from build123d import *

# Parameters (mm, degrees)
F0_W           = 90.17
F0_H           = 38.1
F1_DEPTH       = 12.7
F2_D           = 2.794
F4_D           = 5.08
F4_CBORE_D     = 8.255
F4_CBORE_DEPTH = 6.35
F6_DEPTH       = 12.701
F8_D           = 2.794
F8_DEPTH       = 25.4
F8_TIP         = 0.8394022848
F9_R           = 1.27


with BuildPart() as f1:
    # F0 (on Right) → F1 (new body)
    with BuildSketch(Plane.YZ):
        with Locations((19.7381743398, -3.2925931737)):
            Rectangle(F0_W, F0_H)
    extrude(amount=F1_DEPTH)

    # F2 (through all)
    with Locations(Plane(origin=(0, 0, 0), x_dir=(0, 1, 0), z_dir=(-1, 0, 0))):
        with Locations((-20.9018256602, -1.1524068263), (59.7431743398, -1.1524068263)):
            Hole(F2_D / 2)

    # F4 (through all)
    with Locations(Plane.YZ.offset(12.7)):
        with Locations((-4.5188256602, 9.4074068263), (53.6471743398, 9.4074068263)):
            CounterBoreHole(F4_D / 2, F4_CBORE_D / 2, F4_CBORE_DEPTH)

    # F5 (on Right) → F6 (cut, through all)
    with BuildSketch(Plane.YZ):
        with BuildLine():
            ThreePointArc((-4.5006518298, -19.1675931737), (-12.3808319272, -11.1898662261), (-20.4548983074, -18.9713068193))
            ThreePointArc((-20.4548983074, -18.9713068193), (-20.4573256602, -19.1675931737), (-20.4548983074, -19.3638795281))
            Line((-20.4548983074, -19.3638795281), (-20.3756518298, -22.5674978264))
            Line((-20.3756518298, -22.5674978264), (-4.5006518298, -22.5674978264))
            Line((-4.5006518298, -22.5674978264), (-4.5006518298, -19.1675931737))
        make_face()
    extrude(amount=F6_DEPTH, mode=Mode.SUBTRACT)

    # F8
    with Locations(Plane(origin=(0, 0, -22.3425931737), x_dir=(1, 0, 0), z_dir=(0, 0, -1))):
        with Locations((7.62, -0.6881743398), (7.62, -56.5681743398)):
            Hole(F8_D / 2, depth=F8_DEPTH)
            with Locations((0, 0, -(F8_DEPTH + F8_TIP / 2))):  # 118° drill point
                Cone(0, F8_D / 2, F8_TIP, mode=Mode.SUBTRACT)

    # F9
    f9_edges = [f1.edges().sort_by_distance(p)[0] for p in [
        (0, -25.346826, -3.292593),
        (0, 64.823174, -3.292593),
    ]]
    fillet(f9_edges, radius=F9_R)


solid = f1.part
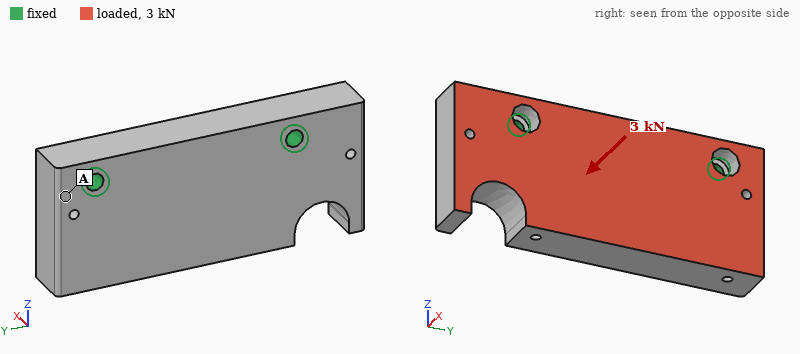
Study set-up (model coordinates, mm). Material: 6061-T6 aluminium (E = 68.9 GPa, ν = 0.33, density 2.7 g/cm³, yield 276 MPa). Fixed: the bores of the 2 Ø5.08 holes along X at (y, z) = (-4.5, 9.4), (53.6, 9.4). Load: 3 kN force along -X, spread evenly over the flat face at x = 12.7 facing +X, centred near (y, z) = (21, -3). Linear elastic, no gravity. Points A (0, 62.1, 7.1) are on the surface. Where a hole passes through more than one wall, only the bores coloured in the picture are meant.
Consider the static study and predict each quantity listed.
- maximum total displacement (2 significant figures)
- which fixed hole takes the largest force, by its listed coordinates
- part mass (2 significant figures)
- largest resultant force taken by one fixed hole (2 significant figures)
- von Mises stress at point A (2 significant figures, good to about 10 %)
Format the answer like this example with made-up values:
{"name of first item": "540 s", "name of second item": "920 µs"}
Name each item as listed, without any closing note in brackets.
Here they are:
{"maximum total displacement": "70 µm", "which fixed hole takes the largest force, by its listed coordinates": "(-4.5, 9.4)", "part mass": "110 g", "largest resultant force taken by one fixed hole": "1.7 kN", "von Mises stress at point A": "18 MPa"}
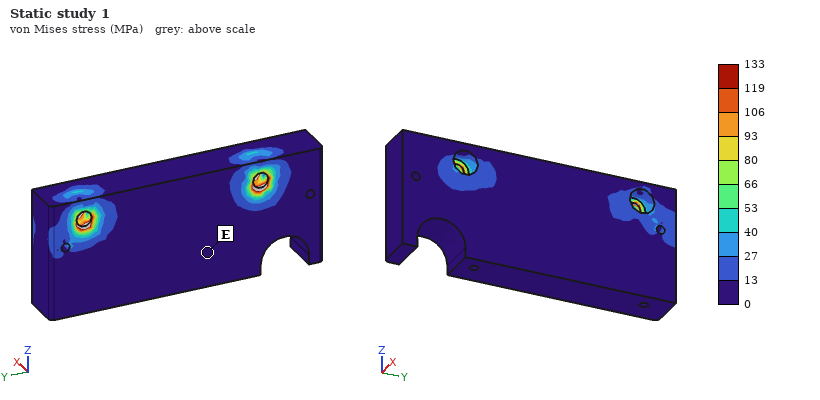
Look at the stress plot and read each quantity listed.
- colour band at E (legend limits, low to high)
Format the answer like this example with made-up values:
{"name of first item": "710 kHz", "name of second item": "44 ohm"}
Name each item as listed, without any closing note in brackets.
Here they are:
{"colour band at E": "0 to 13 MPa"}
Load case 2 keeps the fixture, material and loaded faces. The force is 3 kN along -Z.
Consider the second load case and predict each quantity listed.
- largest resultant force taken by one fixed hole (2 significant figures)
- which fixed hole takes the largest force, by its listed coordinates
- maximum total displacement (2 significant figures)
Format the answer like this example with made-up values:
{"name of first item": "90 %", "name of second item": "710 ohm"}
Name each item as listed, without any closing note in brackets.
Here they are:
{"largest resultant force taken by one fixed hole": "1.7 kN", "which fixed hole takes the largest force, by its listed coordinates": "(-4.5, 9.4)", "maximum total displacement": "50 µm"}
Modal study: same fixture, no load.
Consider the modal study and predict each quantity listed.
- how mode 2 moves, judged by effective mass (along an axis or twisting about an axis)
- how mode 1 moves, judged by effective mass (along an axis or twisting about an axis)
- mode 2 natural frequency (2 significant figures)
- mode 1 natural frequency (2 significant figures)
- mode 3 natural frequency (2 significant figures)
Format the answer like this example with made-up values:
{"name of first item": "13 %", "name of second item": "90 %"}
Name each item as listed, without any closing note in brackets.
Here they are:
{"how mode 2 moves, judged by effective mass": "twisting about Z", "how mode 1 moves, judged by effective mass": "along X", "mode 2 natural frequency": "7600 Hz", "mode 1 natural frequency": "3900 Hz", "mode 3 natural frequency": "10 kHz"}
